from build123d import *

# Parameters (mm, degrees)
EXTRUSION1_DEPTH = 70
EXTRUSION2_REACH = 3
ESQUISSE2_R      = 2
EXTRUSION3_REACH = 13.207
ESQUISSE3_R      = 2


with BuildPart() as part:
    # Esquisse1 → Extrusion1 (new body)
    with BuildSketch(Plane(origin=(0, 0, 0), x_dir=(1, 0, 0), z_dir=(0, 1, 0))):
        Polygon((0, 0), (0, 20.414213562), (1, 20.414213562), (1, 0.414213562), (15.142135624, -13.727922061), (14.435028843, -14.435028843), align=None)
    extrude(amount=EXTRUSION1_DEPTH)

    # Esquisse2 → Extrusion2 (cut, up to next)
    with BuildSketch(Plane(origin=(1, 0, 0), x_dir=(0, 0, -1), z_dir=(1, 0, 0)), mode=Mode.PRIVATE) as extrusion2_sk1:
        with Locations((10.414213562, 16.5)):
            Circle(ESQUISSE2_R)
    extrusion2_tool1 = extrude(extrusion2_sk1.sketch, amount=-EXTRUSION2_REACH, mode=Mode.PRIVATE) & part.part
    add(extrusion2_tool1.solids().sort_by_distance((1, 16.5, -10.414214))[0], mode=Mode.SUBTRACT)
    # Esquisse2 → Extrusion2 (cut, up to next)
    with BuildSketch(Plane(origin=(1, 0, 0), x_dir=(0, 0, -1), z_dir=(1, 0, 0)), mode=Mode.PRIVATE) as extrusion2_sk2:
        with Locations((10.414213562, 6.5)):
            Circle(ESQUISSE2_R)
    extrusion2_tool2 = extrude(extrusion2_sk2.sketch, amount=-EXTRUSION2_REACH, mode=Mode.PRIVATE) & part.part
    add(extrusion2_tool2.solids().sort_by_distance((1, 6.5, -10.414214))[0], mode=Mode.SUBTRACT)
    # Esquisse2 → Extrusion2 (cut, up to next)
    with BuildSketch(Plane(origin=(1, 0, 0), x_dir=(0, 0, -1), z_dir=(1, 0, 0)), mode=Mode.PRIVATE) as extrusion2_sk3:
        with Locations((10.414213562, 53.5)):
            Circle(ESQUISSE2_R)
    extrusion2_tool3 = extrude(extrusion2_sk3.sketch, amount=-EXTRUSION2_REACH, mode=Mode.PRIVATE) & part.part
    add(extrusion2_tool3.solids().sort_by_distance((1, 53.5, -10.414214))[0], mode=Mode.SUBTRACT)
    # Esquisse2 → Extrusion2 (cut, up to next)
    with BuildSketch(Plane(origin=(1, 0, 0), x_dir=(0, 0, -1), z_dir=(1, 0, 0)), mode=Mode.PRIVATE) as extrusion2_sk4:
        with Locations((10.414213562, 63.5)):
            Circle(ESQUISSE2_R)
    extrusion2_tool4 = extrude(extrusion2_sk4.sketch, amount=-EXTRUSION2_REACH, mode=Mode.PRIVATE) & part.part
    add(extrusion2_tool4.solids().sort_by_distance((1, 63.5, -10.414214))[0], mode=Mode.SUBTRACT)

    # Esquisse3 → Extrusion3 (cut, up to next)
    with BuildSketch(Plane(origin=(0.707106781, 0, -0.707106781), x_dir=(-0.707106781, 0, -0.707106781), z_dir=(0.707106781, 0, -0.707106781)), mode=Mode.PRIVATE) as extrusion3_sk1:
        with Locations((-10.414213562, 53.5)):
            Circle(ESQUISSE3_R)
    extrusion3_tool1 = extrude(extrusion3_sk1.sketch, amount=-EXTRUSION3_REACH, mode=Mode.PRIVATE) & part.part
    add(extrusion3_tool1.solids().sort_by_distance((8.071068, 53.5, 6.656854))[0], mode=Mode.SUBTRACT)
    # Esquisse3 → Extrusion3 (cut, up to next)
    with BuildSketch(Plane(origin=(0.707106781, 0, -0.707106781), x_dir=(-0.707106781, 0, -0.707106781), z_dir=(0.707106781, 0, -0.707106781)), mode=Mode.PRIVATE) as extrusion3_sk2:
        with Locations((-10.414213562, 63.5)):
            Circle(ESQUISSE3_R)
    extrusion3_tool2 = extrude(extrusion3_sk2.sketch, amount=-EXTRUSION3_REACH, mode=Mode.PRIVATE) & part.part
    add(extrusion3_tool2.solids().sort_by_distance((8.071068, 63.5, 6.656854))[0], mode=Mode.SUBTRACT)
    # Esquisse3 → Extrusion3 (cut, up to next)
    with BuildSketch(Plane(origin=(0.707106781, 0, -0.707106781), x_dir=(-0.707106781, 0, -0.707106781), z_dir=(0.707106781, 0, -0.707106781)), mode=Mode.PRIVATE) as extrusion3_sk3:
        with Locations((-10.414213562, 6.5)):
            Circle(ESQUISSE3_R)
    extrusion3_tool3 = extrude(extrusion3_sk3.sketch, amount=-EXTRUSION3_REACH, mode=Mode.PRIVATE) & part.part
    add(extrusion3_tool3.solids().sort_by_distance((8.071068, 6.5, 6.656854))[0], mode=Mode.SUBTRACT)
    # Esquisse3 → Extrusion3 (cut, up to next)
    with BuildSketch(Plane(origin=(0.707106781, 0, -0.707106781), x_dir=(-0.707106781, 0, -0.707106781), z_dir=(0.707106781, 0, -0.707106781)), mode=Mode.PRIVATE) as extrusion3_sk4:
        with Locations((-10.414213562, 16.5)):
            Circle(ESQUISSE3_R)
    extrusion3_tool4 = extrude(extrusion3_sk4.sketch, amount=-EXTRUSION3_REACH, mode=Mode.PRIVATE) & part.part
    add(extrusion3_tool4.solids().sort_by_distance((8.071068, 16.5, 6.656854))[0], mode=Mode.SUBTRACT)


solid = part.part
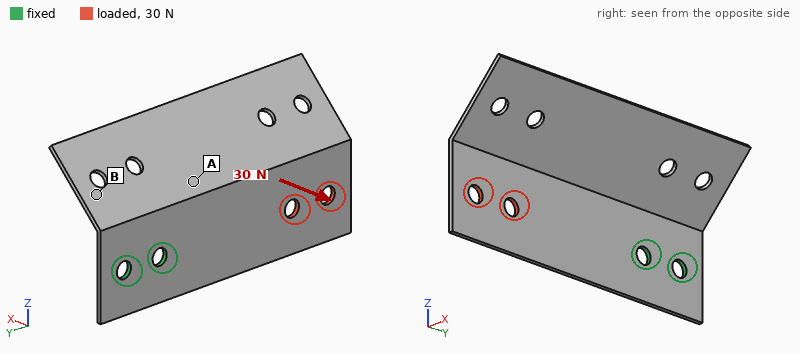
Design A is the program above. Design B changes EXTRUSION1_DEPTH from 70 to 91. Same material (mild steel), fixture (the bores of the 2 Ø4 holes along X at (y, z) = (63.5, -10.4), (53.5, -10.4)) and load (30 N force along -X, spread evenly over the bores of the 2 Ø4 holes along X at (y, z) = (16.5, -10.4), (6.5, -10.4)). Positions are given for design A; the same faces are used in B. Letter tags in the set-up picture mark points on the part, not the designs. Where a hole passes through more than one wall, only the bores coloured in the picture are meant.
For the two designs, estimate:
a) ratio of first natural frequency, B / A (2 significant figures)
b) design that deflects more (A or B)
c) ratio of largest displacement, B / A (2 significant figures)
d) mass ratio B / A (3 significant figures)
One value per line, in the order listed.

1.1
A
0.92
1.31
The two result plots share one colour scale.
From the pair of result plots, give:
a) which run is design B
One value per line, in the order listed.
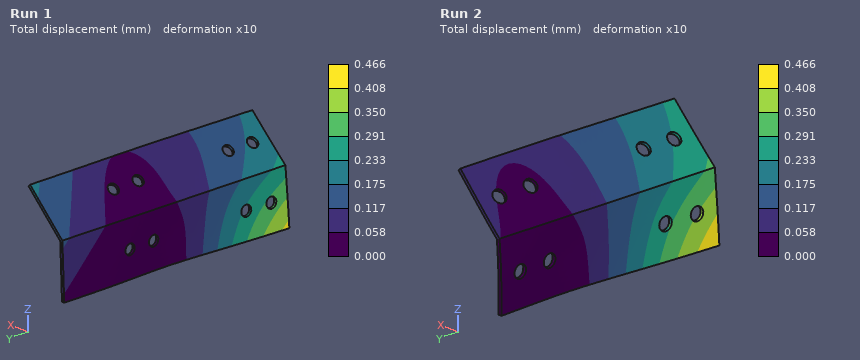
Run 1
